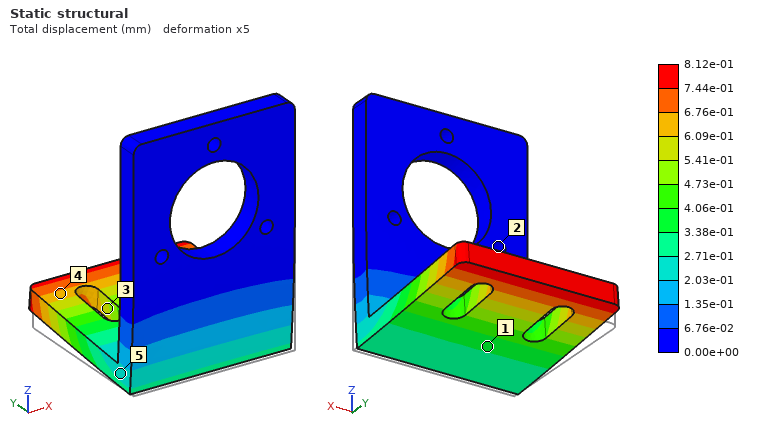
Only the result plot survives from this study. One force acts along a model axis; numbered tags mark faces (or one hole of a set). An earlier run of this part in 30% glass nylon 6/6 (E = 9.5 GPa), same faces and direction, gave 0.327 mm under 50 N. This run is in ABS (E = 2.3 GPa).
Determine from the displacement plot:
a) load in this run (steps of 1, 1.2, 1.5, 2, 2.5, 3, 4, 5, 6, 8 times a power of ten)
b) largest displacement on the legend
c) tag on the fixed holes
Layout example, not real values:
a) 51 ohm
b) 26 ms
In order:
a) 30 N
b) 8.12e-01 mm
c) 2
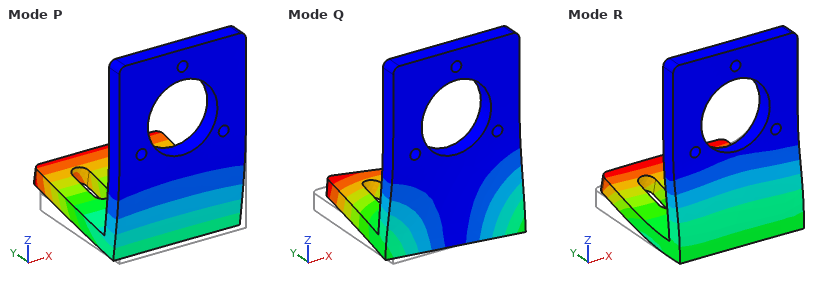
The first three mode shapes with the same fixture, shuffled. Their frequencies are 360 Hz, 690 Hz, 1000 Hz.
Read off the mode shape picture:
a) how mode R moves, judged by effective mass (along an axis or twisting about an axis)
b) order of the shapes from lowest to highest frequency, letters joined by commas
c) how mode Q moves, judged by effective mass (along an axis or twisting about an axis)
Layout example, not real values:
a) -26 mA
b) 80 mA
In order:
a) along Y
b) P, Q, R
c) along X
